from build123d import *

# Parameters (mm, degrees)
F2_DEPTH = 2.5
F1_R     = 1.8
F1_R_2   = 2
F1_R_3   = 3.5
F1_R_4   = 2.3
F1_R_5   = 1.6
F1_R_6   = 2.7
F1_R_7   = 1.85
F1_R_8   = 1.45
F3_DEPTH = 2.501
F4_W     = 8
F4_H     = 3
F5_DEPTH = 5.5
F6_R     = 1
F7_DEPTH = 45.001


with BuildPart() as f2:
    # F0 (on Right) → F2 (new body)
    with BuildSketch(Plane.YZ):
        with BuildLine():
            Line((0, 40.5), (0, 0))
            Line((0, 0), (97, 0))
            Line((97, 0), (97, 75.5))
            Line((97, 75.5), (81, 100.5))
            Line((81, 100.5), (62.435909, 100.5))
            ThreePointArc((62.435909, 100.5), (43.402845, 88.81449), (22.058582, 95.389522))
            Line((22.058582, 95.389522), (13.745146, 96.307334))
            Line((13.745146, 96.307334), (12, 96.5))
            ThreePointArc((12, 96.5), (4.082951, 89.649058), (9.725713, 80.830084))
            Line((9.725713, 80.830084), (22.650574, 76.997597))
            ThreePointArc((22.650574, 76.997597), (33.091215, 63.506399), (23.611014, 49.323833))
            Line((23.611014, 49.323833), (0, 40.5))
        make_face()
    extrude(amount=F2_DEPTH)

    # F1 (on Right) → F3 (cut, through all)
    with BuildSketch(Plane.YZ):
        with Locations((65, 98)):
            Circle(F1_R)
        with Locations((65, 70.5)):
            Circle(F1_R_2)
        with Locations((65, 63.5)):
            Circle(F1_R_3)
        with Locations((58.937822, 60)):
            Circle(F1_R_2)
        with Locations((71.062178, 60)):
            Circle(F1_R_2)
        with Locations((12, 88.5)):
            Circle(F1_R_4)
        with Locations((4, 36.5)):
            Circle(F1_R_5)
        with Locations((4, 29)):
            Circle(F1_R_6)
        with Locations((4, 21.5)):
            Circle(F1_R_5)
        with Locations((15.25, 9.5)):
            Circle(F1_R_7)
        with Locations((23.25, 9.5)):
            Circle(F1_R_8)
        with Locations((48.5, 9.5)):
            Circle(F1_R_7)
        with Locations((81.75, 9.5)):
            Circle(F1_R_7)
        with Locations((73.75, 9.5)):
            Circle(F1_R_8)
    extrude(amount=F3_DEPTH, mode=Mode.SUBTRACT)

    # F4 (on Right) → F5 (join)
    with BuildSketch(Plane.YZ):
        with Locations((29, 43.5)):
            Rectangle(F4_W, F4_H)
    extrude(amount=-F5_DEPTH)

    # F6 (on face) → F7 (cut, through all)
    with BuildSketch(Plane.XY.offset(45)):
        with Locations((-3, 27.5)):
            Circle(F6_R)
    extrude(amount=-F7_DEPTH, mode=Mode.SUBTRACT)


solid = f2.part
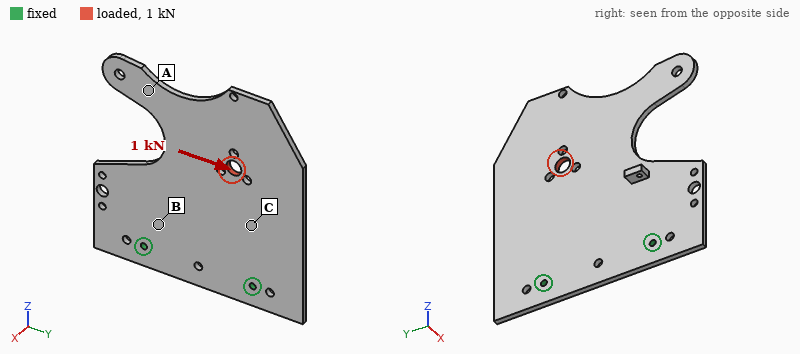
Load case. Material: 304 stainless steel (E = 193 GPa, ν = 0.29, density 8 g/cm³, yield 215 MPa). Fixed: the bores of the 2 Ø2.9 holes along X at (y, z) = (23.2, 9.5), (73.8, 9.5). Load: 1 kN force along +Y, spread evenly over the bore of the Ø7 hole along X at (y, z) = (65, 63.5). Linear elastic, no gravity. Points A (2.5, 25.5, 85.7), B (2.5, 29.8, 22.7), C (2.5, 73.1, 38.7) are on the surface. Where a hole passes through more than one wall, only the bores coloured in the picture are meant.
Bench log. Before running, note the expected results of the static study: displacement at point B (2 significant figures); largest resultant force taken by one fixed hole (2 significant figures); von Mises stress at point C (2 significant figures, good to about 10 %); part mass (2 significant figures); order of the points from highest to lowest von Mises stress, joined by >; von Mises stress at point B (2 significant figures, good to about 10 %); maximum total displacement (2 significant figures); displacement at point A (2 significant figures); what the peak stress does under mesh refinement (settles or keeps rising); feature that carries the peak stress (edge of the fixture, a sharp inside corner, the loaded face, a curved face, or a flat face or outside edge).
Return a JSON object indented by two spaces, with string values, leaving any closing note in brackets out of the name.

{
  "displacement at point B": "2.7 µm",
  "largest resultant force taken by one fixed hole": "1.2 kN",
  "von Mises stress at point C": "11 MPa",
  "part mass": "160 g",
  "order of the points from highest to lowest von Mises stress, joined by >": "B > C > A",
  "von Mises stress at point B": "20 MPa",
  "maximum total displacement": "18 µm",
  "displacement at point A": "15 µm",
  "what the peak stress does under mesh refinement": "keeps rising",
  "feature that carries the peak stress": "edge of the fixture"
}
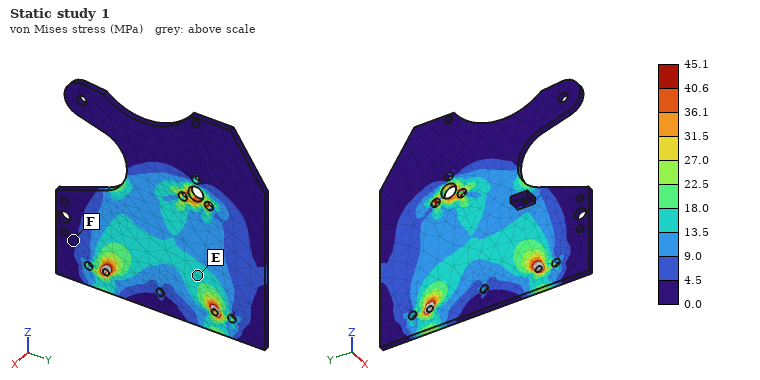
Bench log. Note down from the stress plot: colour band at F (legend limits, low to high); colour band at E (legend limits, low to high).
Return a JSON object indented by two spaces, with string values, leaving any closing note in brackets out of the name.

{
  "colour band at F": "0.0 to 4.5 MPa",
  "colour band at E": "13.5 to 18.0 MPa"
}
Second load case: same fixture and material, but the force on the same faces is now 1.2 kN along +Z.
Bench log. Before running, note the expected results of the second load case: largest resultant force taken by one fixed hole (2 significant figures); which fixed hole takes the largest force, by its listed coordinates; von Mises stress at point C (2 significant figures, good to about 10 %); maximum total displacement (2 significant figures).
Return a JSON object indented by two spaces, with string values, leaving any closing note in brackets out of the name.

{
  "largest resultant force taken by one fixed hole": "990 N",
  "which fixed hole takes the largest force, by its listed coordinates": "(73.8, 9.5)",
  "von Mises stress at point C": "12 MPa",
  "maximum total displacement": "6.0 µm"
}
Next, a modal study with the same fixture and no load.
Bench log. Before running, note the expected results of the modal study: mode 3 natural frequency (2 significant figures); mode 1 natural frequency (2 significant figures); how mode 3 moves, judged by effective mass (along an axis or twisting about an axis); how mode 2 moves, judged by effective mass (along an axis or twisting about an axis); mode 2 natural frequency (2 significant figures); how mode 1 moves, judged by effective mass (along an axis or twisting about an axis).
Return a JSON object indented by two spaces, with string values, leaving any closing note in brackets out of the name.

{
  "mode 3 natural frequency": "1400 Hz",
  "mode 1 natural frequency": "260 Hz",
  "how mode 3 moves, judged by effective mass": "along X",
  "how mode 2 moves, judged by effective mass": "twisting about Z",
  "mode 2 natural frequency": "610 Hz",
  "how mode 1 moves, judged by effective mass": "along X"
}
